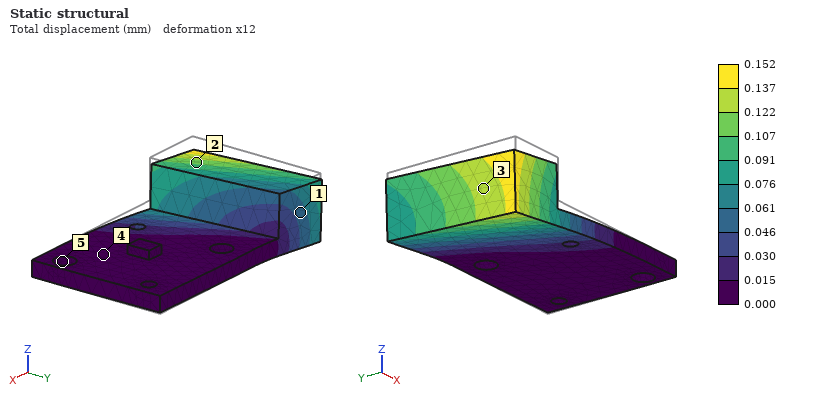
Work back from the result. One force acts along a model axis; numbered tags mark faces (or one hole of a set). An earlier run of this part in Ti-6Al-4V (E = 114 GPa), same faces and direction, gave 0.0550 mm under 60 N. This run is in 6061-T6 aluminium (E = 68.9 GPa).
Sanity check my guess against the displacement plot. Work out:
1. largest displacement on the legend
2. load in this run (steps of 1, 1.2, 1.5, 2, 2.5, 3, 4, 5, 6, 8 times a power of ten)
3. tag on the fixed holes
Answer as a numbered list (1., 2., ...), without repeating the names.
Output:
1. 0.152 mm
2. 100 N
3. 5
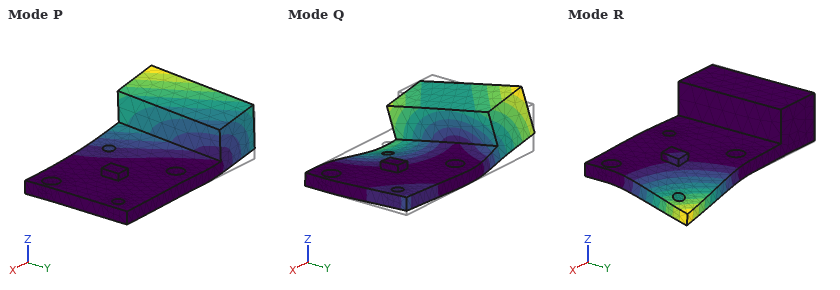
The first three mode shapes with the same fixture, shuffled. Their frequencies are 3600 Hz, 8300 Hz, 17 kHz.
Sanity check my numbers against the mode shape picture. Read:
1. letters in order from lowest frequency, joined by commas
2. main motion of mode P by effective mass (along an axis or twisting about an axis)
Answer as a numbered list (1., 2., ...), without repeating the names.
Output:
1. P, Q, R
2. along Z
